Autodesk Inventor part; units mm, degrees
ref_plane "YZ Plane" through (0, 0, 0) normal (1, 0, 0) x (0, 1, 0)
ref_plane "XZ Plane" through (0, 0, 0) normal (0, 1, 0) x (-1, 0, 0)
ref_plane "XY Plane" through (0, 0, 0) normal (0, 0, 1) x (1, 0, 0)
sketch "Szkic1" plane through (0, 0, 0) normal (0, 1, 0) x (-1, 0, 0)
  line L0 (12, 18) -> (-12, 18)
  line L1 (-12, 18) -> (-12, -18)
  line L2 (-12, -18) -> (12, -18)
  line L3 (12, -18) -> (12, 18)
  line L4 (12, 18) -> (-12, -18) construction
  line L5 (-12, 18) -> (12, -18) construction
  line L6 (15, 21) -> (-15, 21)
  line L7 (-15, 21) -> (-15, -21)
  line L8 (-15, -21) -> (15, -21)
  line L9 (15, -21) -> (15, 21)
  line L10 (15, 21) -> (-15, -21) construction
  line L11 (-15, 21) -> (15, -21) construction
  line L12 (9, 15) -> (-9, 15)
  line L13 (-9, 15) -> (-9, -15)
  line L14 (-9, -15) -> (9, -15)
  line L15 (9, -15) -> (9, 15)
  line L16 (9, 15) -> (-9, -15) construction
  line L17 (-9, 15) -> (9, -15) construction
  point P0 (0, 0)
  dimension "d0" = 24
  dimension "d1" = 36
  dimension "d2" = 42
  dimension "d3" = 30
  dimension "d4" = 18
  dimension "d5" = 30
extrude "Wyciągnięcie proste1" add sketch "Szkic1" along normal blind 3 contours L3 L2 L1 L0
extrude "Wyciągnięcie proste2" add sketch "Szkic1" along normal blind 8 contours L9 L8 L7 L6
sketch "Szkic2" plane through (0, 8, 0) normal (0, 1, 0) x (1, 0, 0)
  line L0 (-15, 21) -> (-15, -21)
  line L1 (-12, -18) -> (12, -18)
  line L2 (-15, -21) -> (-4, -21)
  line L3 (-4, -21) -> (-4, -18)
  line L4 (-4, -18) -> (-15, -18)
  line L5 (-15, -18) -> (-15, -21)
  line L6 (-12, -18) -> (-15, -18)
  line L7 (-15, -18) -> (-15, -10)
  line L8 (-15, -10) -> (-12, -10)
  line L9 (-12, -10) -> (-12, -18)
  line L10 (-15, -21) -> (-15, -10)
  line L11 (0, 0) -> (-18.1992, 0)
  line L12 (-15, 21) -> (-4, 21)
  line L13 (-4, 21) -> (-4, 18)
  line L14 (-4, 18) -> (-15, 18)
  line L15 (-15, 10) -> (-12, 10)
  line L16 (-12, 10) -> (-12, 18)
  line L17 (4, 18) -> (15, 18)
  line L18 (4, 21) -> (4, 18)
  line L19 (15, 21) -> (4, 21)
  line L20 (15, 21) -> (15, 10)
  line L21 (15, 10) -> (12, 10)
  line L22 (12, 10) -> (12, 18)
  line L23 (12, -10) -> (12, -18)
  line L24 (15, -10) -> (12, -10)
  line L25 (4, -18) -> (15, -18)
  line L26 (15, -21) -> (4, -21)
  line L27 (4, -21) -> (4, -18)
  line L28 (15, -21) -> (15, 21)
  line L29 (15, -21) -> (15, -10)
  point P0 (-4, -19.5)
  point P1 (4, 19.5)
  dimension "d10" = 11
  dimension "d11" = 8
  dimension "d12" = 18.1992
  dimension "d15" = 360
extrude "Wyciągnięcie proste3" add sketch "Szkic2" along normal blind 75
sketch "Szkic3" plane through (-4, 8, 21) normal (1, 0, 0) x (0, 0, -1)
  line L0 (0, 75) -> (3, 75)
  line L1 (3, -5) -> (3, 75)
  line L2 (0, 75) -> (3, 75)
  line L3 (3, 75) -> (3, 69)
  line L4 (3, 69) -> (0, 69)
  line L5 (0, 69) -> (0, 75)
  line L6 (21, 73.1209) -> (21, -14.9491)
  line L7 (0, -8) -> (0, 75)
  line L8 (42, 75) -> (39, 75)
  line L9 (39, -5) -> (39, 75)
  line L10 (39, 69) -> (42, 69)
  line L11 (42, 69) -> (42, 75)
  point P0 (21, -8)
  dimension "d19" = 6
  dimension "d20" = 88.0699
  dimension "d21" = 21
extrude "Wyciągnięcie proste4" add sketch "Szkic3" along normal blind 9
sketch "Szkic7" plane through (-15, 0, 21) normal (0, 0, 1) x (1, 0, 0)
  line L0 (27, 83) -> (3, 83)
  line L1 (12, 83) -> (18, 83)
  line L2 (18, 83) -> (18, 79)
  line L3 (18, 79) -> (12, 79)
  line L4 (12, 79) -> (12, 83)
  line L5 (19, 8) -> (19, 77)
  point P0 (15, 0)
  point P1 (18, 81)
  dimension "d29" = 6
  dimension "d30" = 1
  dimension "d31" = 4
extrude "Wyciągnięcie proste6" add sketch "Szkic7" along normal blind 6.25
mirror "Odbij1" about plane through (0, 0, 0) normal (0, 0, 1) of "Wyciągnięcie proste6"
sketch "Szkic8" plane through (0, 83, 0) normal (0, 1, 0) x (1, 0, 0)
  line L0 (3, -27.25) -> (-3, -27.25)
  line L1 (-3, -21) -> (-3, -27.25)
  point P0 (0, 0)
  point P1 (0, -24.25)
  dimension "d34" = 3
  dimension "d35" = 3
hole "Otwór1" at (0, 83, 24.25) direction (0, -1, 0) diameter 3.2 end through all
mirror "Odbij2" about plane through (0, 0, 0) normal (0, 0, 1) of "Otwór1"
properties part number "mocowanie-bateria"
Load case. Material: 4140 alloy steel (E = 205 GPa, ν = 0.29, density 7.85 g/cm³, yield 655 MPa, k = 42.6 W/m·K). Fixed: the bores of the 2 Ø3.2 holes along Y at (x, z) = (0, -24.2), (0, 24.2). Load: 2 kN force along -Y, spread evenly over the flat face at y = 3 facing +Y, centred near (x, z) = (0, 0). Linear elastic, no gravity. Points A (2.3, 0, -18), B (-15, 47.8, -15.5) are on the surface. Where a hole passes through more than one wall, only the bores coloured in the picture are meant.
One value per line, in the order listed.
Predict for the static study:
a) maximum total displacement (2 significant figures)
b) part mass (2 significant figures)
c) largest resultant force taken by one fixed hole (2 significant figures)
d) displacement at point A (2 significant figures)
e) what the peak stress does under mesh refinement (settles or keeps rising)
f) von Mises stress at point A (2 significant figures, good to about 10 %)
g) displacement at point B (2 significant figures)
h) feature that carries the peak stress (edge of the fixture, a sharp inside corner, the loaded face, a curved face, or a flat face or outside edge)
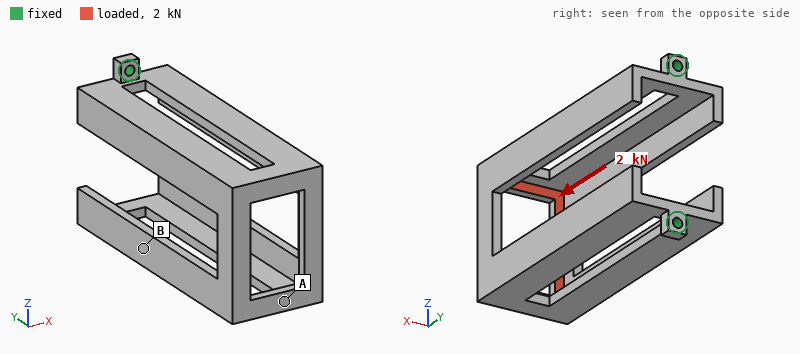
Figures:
23 µm
170 g
1.0 kN
16 µm
keeps rising
35 MPa
18 µm
edge of the fixture
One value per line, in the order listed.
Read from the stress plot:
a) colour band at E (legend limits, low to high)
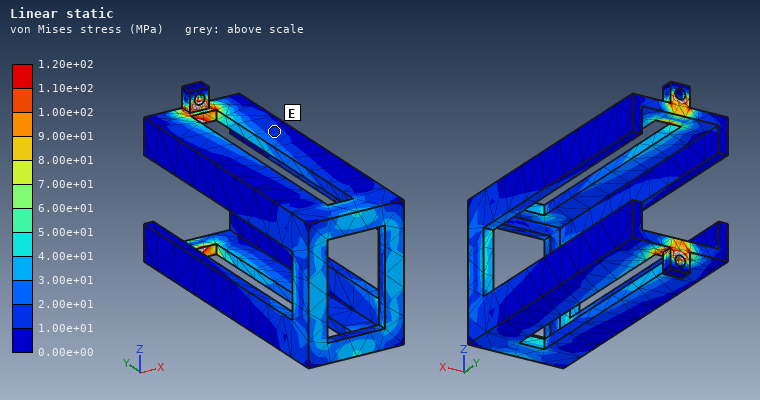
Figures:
1.00e+01 to 2.00e+01 MPa
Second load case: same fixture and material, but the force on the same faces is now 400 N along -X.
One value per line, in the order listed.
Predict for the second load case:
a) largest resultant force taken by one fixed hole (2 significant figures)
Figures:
200 N
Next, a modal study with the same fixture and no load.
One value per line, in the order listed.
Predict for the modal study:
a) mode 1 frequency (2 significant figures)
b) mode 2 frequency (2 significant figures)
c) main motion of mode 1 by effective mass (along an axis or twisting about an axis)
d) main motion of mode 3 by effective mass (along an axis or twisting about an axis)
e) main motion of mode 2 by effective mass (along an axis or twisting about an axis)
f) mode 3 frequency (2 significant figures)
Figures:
410 Hz
880 Hz
along X
twisting about Y
along Z
1200 Hz
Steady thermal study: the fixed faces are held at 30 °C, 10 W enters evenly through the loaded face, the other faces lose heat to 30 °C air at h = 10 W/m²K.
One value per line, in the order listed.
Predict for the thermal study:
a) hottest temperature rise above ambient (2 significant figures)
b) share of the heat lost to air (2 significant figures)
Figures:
66 K
60 %
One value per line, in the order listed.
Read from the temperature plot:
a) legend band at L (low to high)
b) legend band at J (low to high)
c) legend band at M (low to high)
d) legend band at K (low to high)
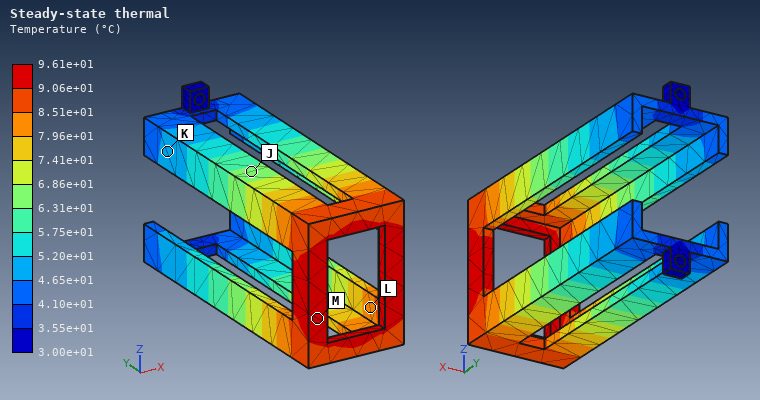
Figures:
7.96e+01 to 8.51e+01 °C
6.31e+01 to 6.86e+01 °C
9.06e+01 to 9.61e+01 °C
4.65e+01 to 5.20e+01 °C
